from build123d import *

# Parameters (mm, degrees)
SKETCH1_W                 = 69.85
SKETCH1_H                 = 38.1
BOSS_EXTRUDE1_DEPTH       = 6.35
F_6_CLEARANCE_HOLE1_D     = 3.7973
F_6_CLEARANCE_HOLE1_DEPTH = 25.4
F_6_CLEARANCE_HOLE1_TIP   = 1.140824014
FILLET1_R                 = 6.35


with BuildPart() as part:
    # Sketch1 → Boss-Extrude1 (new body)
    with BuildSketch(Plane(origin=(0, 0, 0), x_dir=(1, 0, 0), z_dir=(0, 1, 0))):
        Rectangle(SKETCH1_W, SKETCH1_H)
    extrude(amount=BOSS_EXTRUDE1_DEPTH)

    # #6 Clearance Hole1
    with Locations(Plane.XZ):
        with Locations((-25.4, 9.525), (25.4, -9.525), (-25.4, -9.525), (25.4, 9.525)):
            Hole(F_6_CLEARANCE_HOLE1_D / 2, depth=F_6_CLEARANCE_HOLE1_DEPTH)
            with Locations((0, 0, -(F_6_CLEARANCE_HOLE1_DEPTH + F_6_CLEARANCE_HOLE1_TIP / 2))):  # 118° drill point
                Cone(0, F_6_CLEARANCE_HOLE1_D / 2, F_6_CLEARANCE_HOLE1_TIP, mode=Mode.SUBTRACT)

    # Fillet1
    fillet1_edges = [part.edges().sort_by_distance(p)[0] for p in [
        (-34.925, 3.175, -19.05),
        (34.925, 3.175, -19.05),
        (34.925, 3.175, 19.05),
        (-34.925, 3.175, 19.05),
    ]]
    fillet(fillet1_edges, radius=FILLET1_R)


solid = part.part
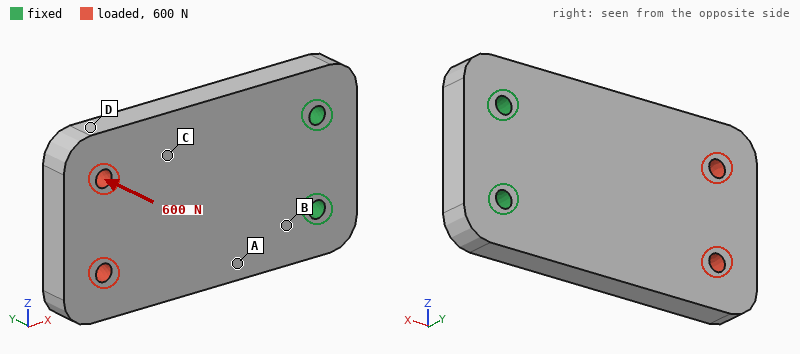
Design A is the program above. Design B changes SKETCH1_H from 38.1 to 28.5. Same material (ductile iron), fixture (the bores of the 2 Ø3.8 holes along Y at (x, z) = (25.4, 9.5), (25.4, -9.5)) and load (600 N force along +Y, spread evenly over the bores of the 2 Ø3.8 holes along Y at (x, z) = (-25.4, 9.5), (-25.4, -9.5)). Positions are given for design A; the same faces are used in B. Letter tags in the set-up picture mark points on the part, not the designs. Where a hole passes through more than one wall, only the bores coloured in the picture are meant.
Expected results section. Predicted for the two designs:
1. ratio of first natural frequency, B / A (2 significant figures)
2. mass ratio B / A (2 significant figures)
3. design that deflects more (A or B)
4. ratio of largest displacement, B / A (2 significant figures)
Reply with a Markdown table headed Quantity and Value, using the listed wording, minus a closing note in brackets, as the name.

| Quantity | Value |
|---|---|
| ratio of first natural frequency, B / A | 1.0 |
| mass ratio B / A | 0.74 |
| design that deflects more | B |
| ratio of largest displacement, B / A | 1.3 |
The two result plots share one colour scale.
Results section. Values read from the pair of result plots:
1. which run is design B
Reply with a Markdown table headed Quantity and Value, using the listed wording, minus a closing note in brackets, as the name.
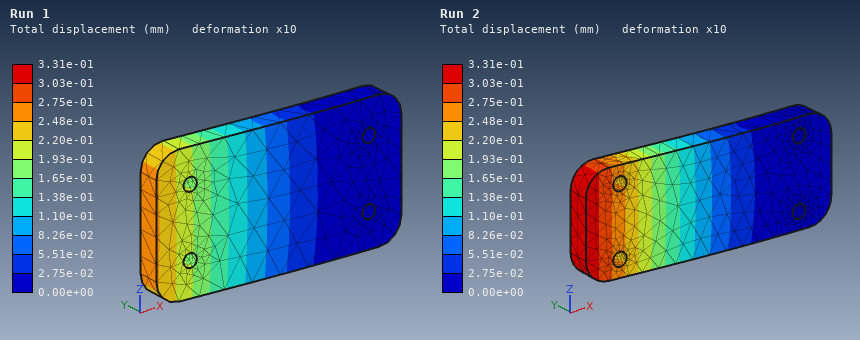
| Quantity | Value |
|---|---|
| which run is design B | Run 2 |
